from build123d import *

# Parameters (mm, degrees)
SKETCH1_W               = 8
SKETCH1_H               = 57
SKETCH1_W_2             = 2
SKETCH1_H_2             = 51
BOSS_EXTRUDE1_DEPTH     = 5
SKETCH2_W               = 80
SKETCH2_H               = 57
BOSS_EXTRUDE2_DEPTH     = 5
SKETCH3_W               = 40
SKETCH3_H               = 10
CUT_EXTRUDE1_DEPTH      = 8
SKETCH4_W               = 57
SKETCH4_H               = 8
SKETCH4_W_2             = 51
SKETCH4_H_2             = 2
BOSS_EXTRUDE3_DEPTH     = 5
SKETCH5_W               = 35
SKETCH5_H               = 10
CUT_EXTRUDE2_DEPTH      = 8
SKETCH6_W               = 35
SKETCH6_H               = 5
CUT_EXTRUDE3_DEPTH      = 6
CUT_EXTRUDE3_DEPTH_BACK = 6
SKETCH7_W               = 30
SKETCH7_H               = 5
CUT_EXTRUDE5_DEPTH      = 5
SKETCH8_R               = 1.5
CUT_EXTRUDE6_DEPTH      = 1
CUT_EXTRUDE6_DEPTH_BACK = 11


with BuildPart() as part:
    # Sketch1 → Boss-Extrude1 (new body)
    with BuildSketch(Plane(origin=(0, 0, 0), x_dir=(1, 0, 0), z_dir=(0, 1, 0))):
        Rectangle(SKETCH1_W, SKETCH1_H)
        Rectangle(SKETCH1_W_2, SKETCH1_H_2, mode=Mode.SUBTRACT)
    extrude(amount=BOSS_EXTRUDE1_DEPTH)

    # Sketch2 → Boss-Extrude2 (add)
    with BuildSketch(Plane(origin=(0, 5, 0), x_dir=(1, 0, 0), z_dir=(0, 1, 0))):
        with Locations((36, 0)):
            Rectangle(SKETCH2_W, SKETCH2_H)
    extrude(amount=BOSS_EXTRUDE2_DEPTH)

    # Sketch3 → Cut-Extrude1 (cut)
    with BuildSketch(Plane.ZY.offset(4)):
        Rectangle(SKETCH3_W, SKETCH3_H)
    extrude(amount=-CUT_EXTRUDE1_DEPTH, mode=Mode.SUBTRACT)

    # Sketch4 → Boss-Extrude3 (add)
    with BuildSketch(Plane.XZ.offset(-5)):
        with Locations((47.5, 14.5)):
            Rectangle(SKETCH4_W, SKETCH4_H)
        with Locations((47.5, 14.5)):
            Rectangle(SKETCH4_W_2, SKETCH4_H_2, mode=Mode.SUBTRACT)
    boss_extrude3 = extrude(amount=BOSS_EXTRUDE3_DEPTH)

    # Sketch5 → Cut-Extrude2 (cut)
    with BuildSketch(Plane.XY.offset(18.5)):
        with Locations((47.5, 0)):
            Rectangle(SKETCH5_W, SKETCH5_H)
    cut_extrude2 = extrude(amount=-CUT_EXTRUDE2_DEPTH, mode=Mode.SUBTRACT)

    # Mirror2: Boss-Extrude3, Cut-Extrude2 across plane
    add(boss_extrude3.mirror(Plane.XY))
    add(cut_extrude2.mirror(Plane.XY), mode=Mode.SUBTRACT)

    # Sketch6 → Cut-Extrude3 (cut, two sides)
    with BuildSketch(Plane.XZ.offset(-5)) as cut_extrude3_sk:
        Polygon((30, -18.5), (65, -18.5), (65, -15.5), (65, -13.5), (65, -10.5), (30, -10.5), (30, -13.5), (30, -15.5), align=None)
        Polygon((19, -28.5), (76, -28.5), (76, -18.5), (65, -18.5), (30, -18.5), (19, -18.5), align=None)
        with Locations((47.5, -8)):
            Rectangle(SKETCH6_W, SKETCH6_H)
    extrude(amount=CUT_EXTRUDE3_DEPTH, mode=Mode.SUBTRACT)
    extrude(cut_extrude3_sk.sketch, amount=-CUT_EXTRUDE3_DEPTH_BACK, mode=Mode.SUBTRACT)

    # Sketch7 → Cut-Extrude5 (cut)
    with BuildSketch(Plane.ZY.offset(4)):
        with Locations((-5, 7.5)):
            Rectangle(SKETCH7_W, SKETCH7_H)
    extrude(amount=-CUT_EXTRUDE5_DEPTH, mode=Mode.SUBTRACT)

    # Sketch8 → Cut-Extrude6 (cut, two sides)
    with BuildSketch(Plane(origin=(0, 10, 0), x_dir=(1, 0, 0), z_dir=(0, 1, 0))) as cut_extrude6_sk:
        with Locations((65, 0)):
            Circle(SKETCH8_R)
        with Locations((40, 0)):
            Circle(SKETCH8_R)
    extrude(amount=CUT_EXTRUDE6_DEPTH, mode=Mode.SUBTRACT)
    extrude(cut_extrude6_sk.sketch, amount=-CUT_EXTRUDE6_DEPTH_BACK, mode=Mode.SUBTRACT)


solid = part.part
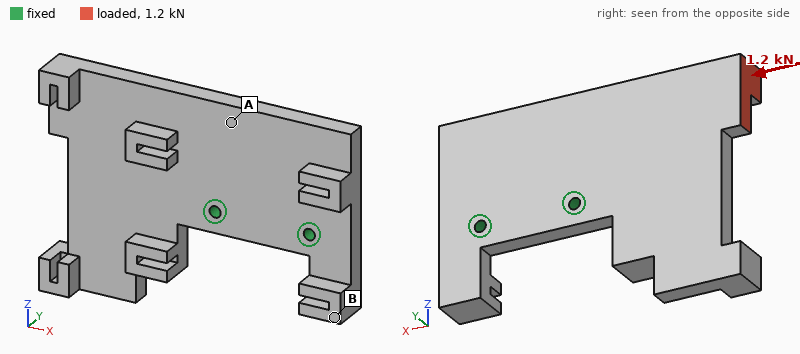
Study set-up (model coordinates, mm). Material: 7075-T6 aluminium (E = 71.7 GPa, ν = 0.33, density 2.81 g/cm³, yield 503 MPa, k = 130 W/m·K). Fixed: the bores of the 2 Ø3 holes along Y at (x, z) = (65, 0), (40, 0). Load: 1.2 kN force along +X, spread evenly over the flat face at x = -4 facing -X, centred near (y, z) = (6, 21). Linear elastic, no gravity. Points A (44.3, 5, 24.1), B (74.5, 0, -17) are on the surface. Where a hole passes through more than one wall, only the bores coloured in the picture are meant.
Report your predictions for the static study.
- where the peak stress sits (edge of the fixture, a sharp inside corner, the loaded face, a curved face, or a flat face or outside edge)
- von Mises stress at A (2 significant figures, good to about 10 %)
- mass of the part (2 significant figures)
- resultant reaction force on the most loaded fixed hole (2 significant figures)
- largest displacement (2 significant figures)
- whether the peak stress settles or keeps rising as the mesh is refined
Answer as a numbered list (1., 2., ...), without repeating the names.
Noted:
1. edge of the fixture
2. 20 MPa
3. 53 g
4. 1.1 kN
5. 0.11 mm
6. keeps rising
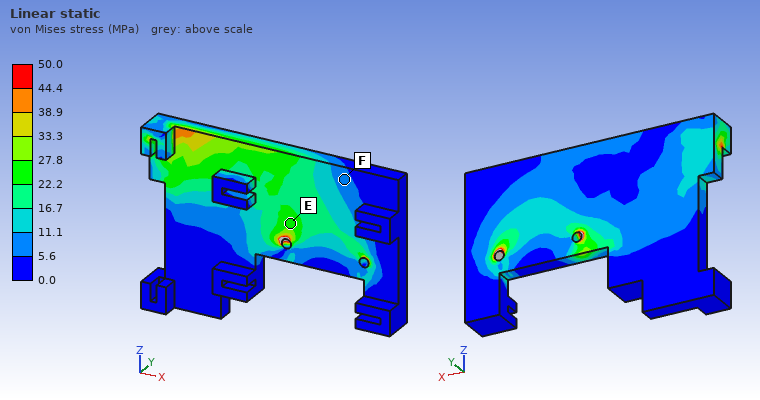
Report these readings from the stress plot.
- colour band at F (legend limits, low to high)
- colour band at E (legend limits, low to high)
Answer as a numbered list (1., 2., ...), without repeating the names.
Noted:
1. 5.6 to 11.1 MPa
2. 22.2 to 27.8 MPa
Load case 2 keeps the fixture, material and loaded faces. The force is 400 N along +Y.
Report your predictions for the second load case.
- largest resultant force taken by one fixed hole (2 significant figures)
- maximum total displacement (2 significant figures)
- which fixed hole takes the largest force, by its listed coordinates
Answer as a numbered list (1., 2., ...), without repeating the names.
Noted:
1. 770 N
2. 0.74 mm
3. (40, 0)
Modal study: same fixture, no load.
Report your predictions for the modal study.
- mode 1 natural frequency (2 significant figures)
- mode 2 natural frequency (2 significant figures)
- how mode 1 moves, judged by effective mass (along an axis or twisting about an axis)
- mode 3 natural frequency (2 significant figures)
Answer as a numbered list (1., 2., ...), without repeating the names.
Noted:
1. 1500 Hz
2. 1900 Hz
3. along Y
4. 4700 Hz
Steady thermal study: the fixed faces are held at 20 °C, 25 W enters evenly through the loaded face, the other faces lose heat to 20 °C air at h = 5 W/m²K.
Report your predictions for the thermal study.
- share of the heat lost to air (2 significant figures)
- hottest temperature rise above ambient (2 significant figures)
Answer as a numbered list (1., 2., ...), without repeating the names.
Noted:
1. 3.9 %
2. 74 K
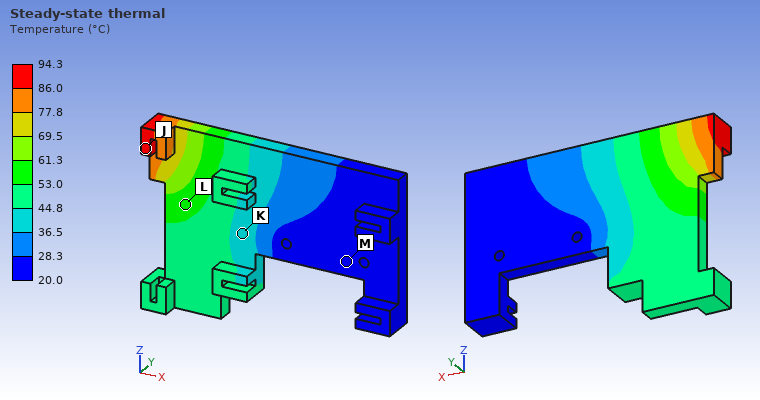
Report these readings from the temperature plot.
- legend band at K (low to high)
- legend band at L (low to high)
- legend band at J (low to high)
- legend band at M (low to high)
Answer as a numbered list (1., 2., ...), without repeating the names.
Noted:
1. 36.5 to 44.8 °C
2. 53.0 to 61.3 °C
3. 86.0 to 94.3 °C
4. 20.0 to 28.3 °C
